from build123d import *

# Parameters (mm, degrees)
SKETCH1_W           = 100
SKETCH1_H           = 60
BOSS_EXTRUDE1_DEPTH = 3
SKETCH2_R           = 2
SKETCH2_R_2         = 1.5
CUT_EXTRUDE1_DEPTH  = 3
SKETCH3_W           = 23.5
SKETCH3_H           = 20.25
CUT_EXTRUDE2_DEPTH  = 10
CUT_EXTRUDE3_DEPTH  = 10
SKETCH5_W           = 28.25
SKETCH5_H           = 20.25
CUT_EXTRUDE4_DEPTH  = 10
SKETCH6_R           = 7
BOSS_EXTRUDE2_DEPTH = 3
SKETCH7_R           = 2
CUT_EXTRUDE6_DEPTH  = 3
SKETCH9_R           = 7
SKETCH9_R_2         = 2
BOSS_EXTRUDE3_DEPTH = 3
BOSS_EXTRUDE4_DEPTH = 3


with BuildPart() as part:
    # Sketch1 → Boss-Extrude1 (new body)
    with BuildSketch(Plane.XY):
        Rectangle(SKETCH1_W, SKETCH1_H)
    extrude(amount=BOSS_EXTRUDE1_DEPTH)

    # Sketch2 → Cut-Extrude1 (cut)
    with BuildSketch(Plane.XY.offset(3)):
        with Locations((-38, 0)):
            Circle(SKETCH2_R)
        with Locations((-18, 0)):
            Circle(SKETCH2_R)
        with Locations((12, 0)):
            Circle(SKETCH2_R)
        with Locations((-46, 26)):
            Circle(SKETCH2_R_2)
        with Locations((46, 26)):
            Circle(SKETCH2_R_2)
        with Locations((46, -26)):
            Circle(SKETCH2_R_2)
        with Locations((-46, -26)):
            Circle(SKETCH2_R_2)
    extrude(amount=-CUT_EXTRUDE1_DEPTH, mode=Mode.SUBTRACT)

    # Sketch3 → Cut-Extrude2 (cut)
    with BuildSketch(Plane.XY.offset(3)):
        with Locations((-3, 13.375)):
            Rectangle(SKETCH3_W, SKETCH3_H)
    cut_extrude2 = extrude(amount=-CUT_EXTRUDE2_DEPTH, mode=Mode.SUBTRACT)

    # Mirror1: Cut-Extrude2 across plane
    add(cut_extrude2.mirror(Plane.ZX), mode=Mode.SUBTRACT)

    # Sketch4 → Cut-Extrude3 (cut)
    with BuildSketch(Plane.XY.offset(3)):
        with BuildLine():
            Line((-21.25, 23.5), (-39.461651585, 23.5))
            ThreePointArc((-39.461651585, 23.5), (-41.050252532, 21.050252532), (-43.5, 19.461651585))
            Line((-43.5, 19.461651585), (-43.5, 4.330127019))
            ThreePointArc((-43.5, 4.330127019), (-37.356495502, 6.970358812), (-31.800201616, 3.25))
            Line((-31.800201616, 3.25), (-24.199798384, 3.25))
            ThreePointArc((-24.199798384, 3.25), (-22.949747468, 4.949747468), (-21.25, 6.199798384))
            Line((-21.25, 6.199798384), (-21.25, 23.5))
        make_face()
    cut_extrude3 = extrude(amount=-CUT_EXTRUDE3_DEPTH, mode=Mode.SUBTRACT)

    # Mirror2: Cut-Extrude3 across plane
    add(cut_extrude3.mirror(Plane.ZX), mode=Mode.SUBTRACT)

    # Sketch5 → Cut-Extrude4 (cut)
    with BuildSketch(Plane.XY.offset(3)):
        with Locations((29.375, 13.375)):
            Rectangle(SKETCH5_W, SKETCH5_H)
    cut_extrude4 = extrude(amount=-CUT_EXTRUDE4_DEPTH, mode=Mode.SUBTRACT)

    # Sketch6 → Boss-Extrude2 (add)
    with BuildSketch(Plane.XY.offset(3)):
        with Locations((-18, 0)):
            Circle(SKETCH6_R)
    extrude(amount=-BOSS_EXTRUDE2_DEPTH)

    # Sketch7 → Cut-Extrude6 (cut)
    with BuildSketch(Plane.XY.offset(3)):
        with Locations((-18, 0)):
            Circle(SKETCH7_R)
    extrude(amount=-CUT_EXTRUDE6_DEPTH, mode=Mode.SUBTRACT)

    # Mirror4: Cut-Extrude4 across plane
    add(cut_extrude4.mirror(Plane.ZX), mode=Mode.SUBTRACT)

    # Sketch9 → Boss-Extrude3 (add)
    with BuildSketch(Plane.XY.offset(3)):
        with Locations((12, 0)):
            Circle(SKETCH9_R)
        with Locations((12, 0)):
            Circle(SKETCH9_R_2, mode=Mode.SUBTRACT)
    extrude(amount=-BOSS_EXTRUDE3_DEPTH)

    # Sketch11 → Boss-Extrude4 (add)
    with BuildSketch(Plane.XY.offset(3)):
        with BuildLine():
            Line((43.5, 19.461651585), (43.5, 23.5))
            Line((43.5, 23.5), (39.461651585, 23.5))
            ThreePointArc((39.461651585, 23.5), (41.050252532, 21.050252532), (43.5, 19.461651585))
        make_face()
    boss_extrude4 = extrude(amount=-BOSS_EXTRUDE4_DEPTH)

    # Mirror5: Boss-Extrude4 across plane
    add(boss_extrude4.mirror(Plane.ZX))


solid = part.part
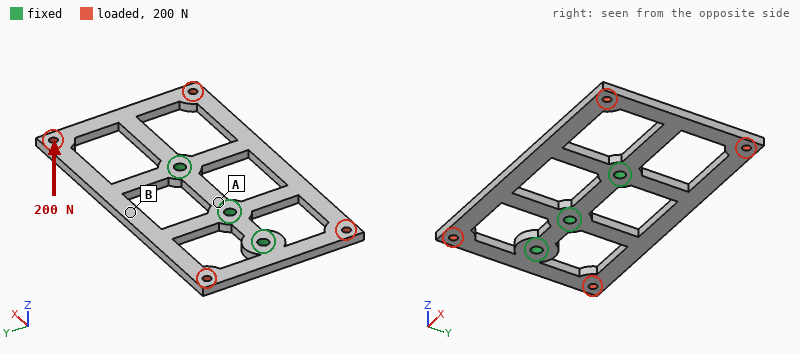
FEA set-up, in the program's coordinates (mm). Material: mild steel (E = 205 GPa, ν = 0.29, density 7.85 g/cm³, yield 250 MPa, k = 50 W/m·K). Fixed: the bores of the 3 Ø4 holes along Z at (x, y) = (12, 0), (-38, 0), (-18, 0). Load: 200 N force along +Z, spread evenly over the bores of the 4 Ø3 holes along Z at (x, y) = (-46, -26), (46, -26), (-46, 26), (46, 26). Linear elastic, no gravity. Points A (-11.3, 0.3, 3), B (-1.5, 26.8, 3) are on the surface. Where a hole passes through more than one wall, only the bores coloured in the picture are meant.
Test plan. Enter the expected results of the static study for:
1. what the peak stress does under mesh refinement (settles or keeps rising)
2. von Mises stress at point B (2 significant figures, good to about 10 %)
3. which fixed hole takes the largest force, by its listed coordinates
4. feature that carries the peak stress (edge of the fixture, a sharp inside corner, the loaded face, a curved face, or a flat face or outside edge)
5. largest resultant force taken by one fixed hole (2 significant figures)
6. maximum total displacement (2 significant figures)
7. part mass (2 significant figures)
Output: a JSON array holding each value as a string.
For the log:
["keeps rising", "34 MPa", "(12, 0)", "edge of the fixture", "130 N", "0.26 mm", "73 g"]
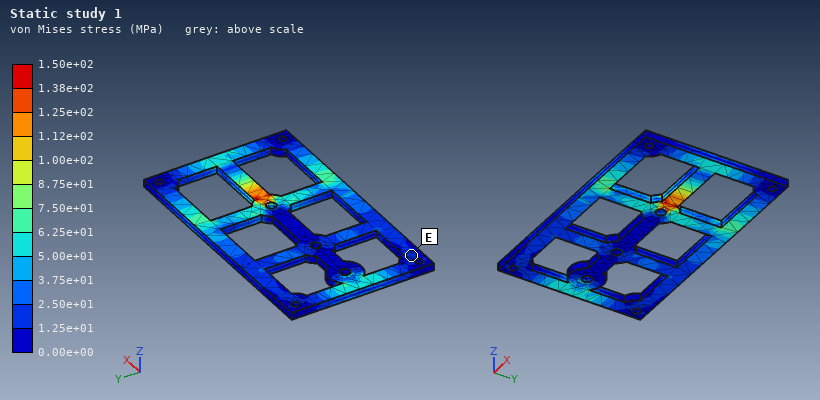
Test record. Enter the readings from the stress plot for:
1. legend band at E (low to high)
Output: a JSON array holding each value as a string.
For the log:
["1.25e+01 to 2.50e+01 MPa"]
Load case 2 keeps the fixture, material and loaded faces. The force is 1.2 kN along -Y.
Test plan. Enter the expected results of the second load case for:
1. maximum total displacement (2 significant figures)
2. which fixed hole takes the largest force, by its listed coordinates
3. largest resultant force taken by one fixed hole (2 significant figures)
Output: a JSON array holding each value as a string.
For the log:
["69 µm", "(12, 0)", "840 N"]
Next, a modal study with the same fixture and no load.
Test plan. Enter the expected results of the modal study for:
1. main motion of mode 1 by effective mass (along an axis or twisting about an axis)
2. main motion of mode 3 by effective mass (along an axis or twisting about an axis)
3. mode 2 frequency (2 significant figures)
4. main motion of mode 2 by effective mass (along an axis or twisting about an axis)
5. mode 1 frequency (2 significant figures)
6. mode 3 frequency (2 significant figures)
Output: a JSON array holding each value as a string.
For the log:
["along Z", "along Z", "1300 Hz", "twisting about X", "1000 Hz", "1900 Hz"]
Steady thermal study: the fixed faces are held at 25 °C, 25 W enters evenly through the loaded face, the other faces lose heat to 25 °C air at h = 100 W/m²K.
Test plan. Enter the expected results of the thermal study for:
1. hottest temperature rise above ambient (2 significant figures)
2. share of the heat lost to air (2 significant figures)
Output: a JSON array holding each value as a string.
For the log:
["75 K", "78 %"]
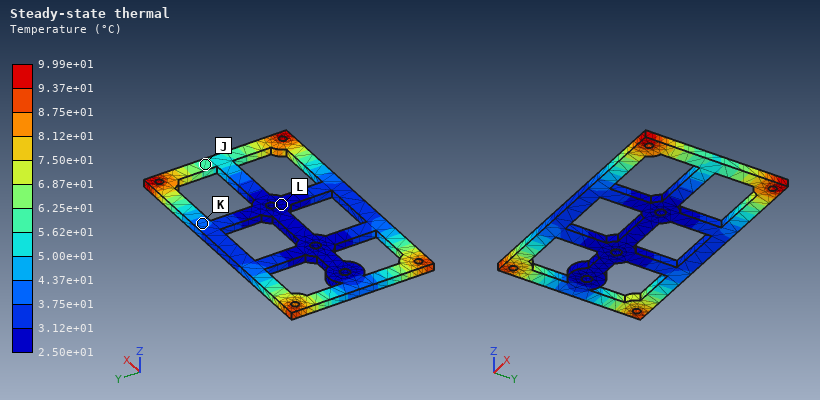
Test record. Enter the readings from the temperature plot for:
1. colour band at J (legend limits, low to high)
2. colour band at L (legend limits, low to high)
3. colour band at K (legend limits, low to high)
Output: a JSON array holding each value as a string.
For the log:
["5.62e+01 to 6.25e+01 °C", "2.50e+01 to 3.12e+01 °C", "3.75e+01 to 4.37e+01 °C"]
